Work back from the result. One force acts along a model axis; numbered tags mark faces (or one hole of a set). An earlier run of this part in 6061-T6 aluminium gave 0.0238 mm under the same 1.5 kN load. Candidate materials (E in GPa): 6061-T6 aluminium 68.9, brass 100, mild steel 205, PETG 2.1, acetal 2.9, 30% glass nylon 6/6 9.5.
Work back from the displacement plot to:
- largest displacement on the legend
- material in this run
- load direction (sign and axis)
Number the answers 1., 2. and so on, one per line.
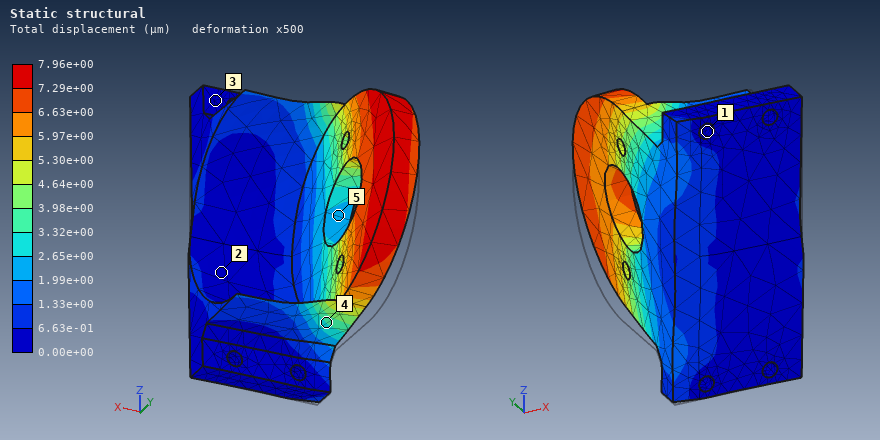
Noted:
1. 7.96e+00 µm
2. mild steel
3. +Z
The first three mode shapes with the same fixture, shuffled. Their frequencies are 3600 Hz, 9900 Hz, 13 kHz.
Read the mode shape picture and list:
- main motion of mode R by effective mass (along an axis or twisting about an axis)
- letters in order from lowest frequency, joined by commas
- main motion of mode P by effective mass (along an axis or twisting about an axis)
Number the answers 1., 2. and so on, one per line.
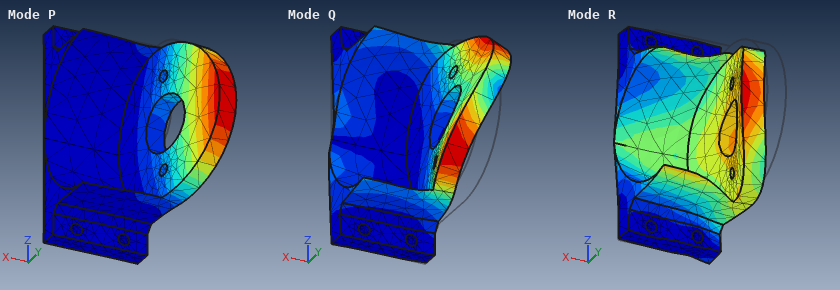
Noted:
1. along Y
2. P, Q, R
3. along X
